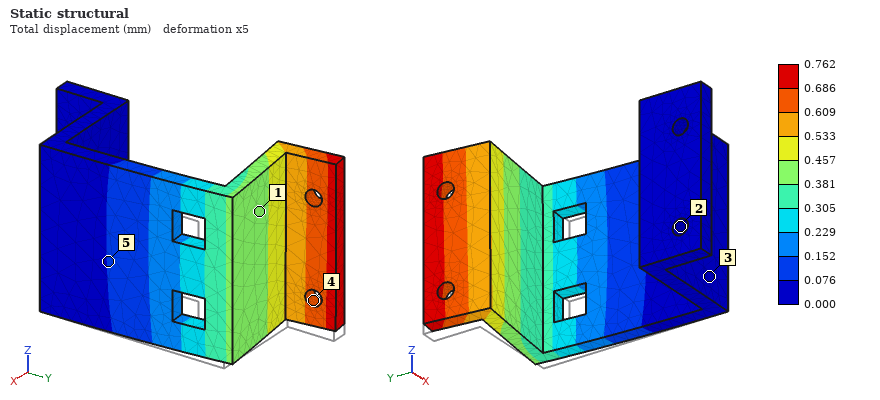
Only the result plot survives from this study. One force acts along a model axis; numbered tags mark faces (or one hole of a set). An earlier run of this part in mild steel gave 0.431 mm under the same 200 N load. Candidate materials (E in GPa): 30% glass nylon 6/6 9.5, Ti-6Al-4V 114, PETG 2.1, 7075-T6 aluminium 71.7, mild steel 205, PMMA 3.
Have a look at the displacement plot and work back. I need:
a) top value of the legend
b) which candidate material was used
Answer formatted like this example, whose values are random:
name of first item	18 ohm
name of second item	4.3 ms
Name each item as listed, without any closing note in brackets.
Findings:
top value of the legend	0.762 mm
which candidate material was used	Ti-6Al-4V
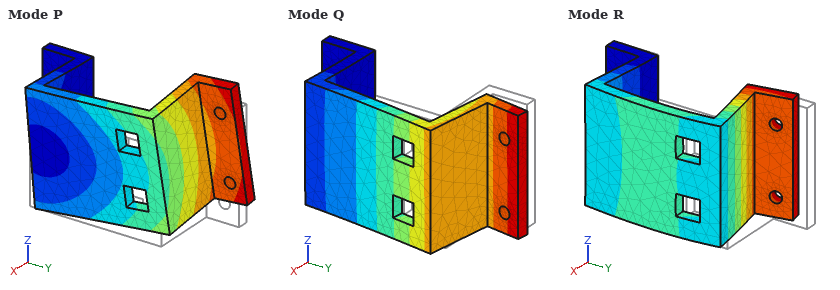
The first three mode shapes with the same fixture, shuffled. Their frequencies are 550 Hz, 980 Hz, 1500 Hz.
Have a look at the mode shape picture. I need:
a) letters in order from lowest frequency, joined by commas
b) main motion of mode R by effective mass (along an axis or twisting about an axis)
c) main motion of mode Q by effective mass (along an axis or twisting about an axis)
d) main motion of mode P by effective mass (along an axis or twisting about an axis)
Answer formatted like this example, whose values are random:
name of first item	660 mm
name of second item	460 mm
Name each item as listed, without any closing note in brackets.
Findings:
letters in order from lowest frequency, joined by commas	Q, P, R
main motion of mode R by effective mass	along Y
main motion of mode Q by effective mass	along X
main motion of mode P by effective mass	along Z
